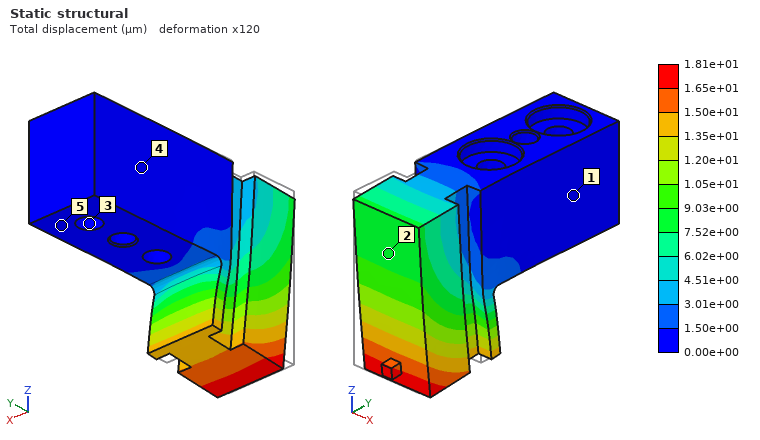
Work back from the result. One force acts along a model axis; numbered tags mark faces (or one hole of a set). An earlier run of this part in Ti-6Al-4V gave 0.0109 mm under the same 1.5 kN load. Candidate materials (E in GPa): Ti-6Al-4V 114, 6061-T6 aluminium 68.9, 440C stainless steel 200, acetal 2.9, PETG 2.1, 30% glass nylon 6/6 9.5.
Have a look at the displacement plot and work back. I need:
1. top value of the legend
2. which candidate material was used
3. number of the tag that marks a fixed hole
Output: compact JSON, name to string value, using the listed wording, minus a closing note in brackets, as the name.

{"top value of the legend": "1.81e+01 µm", "which candidate material was used": "6061-T6 aluminium", "number of the tag that marks a fixed hole": "3"}
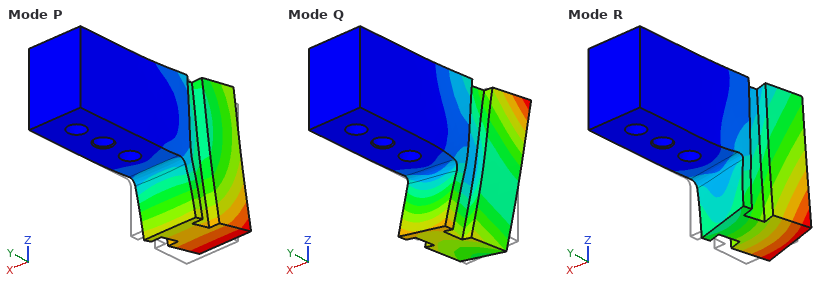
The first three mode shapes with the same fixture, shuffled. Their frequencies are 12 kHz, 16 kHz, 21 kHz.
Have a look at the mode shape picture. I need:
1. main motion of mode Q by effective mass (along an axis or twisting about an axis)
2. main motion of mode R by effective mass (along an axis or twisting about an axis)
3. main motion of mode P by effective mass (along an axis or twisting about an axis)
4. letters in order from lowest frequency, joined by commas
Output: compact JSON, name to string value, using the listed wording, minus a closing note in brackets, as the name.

{"main motion of mode Q by effective mass": "twisting about Y", "main motion of mode R by effective mass": "along X", "main motion of mode P by effective mass": "along Z", "letters in order from lowest frequency, joined by commas": "R, P, Q"}
